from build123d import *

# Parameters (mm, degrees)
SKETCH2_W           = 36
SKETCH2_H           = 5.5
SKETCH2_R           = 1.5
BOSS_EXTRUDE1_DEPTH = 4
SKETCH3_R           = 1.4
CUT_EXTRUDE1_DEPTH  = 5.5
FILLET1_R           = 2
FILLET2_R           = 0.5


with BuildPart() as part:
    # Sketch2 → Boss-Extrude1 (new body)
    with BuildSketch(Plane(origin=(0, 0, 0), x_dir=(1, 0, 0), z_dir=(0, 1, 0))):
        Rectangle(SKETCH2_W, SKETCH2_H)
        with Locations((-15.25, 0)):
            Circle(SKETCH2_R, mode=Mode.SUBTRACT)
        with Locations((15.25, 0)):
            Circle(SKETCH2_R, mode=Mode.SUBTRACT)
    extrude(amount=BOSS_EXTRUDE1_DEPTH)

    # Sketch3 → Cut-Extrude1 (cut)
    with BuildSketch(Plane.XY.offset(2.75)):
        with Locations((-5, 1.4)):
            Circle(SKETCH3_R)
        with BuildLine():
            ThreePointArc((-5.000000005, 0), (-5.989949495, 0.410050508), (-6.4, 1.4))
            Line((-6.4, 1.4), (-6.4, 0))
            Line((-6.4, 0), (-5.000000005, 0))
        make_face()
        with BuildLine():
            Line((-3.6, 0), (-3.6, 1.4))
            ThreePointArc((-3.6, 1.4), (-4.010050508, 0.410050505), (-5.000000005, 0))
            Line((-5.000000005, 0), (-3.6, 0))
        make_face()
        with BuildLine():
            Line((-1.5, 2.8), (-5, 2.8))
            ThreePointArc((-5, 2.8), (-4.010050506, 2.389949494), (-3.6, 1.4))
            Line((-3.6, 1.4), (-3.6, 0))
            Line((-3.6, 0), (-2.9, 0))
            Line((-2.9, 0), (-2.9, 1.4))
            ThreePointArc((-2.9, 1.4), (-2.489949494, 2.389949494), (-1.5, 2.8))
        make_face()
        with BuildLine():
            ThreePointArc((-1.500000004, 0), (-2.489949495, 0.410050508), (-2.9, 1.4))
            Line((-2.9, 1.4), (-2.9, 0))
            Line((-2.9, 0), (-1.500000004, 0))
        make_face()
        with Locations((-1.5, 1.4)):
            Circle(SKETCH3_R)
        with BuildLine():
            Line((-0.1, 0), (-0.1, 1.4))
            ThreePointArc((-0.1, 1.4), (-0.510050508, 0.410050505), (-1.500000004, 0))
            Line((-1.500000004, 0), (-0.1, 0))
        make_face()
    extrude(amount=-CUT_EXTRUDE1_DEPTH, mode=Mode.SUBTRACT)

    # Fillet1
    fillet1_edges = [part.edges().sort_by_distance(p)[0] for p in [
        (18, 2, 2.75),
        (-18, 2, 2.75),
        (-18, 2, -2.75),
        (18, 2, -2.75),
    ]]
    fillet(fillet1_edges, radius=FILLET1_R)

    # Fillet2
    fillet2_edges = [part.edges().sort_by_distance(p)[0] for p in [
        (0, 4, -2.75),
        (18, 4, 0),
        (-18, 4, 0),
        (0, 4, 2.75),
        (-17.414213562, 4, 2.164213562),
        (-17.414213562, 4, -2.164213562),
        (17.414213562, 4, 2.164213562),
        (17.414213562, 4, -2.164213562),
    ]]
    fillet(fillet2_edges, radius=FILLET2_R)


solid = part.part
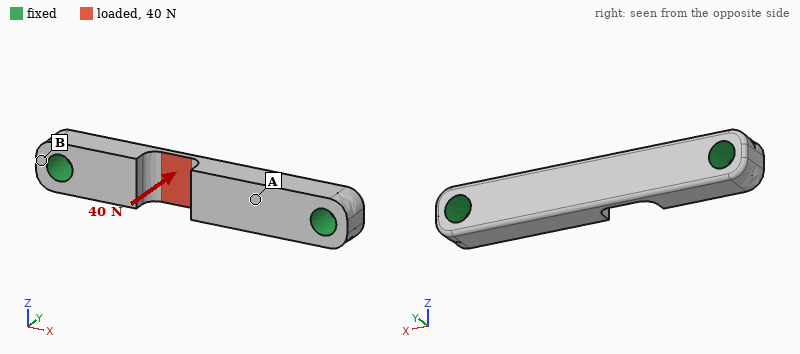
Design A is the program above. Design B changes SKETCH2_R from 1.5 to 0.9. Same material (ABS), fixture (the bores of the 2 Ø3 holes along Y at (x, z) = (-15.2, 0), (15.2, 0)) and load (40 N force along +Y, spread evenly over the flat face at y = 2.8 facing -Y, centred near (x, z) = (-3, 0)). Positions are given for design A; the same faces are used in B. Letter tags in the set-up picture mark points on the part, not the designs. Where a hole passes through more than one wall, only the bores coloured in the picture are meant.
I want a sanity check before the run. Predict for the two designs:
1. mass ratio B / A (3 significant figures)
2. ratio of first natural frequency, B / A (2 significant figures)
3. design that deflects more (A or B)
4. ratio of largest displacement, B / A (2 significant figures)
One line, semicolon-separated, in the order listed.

1.06; 0.91; B; 1.1
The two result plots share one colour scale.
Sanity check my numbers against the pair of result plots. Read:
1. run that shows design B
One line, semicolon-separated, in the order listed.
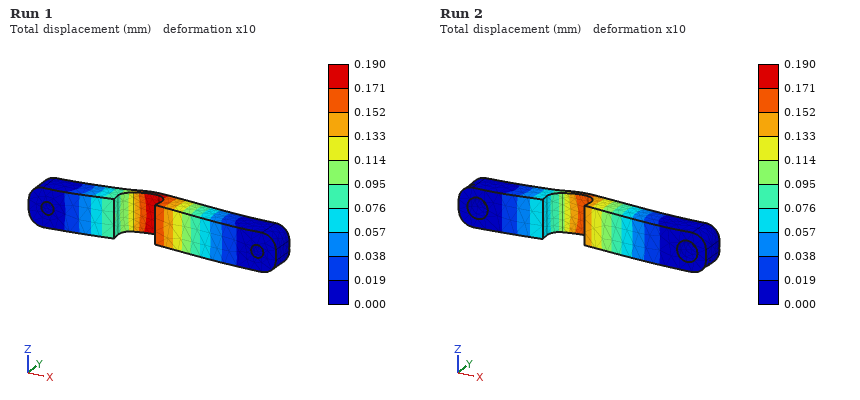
Run 1
